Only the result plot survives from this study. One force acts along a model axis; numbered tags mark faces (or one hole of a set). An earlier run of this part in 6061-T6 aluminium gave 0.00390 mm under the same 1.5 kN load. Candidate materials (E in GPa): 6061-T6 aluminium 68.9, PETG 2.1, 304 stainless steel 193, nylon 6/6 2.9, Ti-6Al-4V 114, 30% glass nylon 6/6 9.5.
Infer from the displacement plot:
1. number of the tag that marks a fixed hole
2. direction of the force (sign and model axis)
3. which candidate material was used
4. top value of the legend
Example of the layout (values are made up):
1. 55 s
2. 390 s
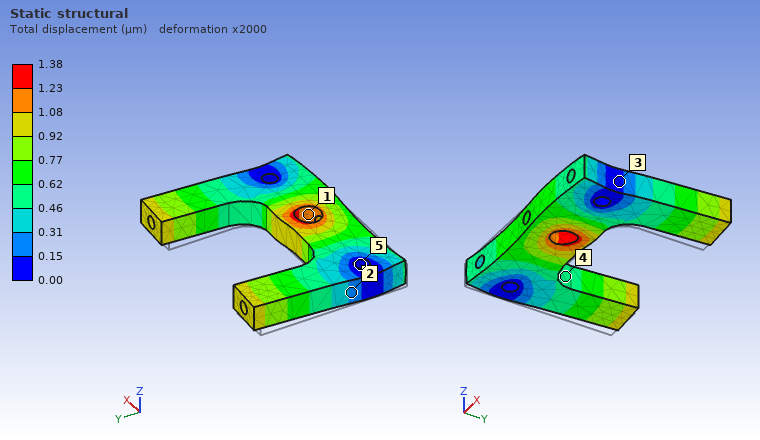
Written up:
1. 5
2. +X
3. 304 stainless steel
4. 1.38 µm
